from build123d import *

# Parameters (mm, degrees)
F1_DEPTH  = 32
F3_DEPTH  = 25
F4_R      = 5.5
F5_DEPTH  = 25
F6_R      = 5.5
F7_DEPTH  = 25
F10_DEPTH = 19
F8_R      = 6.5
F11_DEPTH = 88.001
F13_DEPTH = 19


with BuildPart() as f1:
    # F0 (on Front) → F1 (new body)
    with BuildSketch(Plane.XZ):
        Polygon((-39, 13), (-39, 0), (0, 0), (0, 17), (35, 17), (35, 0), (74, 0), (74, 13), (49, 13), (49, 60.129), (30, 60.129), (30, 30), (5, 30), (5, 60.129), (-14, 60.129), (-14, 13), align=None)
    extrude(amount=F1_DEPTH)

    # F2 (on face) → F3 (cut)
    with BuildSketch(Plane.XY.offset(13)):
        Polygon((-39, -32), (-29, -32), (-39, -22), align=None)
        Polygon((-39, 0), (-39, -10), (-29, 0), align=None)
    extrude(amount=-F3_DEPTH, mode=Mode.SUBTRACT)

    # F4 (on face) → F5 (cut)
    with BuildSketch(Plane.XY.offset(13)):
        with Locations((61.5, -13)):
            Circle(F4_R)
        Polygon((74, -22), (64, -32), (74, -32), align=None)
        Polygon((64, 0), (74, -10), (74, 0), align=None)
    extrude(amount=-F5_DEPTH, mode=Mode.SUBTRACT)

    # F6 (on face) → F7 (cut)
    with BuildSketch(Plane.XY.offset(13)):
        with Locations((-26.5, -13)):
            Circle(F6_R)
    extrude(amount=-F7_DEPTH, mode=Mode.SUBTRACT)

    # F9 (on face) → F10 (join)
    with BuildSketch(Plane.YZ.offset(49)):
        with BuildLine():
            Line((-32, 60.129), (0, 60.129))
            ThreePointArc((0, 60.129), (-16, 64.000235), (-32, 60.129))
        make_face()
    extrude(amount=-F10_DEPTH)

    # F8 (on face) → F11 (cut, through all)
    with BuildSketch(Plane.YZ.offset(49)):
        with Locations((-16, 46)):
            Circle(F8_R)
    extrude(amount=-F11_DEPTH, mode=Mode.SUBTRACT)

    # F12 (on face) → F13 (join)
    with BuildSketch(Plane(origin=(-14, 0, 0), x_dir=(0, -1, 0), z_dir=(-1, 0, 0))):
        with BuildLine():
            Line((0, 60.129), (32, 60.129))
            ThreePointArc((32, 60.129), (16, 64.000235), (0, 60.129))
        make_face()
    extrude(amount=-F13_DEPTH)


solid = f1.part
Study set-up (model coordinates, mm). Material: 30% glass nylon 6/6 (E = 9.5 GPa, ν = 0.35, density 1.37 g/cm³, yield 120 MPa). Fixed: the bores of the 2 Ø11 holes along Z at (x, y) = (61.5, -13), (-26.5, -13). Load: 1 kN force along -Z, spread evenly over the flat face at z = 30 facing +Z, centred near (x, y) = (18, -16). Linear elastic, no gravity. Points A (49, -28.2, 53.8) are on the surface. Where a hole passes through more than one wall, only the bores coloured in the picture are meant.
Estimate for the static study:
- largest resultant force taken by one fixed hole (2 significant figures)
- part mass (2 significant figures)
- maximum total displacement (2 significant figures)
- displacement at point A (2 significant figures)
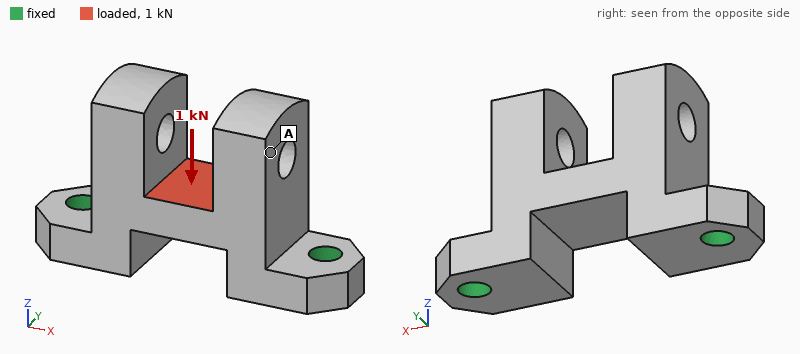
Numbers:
750 N
130 g
38 µm
26 µm
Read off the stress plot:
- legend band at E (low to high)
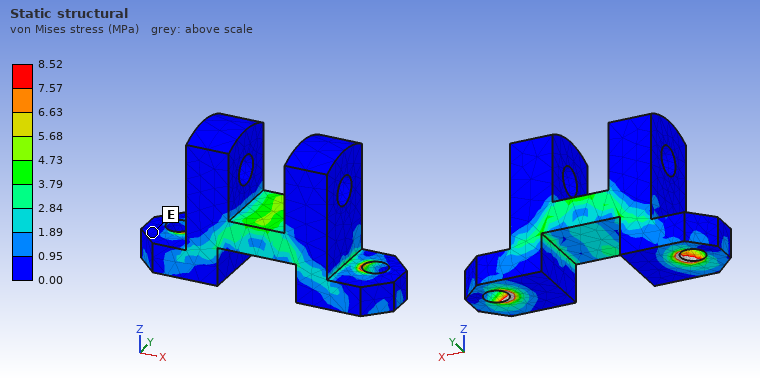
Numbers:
0.00 to 0.95 MPa
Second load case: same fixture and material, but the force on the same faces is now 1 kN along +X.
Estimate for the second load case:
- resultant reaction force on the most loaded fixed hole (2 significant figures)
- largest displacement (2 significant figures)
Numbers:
580 N
19 µm
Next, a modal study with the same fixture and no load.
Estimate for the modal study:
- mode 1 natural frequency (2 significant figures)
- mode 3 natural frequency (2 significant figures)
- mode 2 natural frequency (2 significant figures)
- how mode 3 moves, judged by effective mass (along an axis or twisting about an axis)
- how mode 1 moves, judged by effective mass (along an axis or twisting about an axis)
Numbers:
1400 Hz
3000 Hz
2400 Hz
along X
along Y
